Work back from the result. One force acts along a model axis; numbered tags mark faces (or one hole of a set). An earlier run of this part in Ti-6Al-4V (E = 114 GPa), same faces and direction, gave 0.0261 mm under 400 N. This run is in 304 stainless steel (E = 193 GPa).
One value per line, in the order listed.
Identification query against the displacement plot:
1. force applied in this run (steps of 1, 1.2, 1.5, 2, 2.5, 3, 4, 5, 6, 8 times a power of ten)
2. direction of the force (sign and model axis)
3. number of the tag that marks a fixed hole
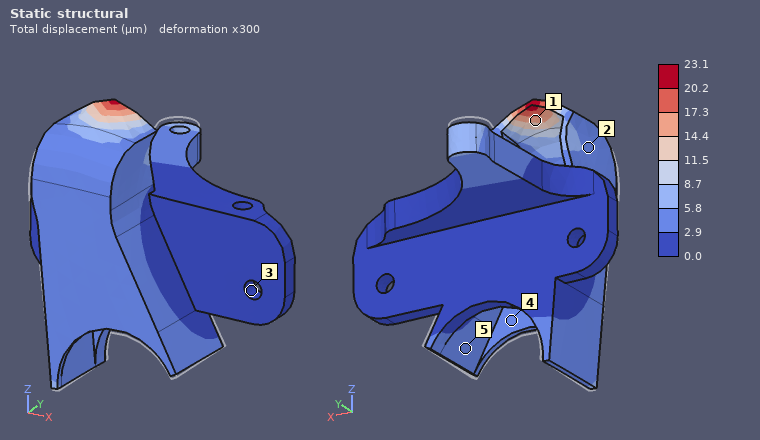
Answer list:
600 N
+Z
3
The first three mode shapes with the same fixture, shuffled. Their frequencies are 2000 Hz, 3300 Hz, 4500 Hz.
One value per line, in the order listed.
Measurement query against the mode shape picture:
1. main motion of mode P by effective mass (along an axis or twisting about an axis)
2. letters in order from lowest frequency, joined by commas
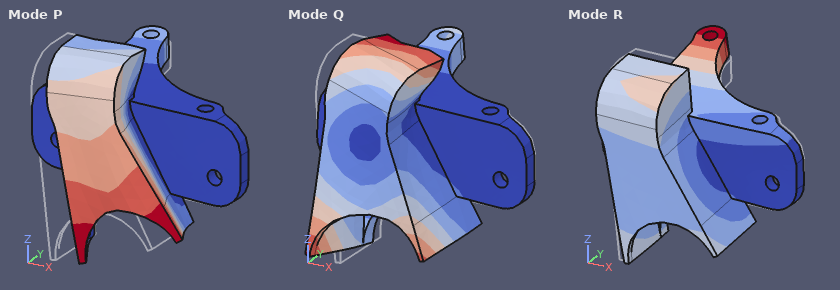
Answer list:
along X
R, P, Q
